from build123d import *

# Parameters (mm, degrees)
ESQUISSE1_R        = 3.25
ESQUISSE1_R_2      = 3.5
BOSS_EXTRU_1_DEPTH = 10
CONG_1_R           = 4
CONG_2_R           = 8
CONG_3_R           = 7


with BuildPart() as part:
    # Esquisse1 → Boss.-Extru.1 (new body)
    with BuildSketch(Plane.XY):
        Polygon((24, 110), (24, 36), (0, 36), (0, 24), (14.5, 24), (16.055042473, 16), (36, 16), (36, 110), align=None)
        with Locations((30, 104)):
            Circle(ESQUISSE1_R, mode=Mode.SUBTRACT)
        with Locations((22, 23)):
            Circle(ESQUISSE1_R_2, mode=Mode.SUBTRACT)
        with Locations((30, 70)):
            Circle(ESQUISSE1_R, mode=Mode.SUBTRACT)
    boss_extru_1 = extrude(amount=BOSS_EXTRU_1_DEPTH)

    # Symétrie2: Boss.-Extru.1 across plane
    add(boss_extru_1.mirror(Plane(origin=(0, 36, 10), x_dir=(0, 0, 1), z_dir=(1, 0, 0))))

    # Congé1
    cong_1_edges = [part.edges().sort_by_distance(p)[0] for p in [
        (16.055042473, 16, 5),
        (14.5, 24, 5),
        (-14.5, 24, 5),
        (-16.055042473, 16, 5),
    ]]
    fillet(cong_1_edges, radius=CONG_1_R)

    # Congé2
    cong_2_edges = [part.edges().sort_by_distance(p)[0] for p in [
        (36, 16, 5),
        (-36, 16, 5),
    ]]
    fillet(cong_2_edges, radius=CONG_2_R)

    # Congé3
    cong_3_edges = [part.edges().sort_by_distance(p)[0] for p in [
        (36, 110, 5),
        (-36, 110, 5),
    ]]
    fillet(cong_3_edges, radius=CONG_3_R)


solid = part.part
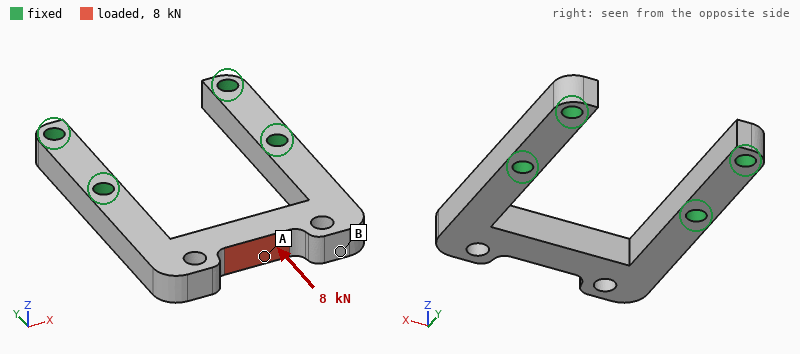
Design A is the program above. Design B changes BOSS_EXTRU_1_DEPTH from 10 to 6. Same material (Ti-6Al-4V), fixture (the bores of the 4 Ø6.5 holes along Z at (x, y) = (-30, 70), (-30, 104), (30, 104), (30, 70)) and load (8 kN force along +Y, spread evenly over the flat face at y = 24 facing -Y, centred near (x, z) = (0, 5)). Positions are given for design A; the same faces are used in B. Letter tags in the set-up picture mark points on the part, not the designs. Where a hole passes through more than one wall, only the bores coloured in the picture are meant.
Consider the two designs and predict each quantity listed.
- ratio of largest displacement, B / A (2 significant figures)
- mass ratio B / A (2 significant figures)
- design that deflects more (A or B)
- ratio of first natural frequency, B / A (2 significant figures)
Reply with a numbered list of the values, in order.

1. 1.7
2. 0.60
3. B
4. 0.62
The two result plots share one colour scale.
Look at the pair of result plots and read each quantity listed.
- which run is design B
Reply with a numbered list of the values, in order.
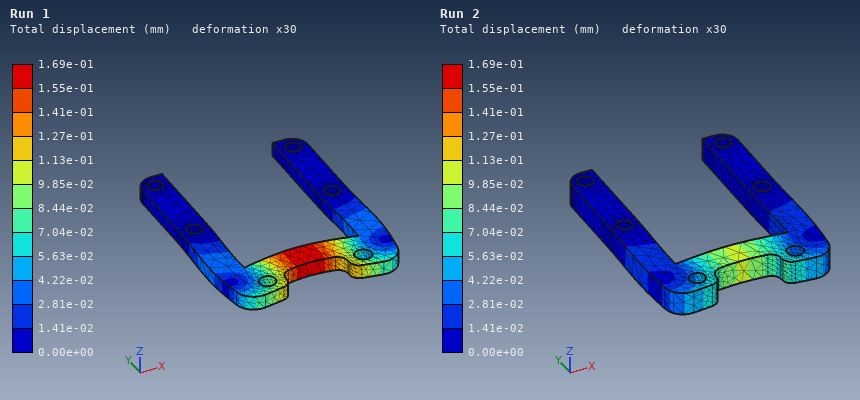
1. Run 1
